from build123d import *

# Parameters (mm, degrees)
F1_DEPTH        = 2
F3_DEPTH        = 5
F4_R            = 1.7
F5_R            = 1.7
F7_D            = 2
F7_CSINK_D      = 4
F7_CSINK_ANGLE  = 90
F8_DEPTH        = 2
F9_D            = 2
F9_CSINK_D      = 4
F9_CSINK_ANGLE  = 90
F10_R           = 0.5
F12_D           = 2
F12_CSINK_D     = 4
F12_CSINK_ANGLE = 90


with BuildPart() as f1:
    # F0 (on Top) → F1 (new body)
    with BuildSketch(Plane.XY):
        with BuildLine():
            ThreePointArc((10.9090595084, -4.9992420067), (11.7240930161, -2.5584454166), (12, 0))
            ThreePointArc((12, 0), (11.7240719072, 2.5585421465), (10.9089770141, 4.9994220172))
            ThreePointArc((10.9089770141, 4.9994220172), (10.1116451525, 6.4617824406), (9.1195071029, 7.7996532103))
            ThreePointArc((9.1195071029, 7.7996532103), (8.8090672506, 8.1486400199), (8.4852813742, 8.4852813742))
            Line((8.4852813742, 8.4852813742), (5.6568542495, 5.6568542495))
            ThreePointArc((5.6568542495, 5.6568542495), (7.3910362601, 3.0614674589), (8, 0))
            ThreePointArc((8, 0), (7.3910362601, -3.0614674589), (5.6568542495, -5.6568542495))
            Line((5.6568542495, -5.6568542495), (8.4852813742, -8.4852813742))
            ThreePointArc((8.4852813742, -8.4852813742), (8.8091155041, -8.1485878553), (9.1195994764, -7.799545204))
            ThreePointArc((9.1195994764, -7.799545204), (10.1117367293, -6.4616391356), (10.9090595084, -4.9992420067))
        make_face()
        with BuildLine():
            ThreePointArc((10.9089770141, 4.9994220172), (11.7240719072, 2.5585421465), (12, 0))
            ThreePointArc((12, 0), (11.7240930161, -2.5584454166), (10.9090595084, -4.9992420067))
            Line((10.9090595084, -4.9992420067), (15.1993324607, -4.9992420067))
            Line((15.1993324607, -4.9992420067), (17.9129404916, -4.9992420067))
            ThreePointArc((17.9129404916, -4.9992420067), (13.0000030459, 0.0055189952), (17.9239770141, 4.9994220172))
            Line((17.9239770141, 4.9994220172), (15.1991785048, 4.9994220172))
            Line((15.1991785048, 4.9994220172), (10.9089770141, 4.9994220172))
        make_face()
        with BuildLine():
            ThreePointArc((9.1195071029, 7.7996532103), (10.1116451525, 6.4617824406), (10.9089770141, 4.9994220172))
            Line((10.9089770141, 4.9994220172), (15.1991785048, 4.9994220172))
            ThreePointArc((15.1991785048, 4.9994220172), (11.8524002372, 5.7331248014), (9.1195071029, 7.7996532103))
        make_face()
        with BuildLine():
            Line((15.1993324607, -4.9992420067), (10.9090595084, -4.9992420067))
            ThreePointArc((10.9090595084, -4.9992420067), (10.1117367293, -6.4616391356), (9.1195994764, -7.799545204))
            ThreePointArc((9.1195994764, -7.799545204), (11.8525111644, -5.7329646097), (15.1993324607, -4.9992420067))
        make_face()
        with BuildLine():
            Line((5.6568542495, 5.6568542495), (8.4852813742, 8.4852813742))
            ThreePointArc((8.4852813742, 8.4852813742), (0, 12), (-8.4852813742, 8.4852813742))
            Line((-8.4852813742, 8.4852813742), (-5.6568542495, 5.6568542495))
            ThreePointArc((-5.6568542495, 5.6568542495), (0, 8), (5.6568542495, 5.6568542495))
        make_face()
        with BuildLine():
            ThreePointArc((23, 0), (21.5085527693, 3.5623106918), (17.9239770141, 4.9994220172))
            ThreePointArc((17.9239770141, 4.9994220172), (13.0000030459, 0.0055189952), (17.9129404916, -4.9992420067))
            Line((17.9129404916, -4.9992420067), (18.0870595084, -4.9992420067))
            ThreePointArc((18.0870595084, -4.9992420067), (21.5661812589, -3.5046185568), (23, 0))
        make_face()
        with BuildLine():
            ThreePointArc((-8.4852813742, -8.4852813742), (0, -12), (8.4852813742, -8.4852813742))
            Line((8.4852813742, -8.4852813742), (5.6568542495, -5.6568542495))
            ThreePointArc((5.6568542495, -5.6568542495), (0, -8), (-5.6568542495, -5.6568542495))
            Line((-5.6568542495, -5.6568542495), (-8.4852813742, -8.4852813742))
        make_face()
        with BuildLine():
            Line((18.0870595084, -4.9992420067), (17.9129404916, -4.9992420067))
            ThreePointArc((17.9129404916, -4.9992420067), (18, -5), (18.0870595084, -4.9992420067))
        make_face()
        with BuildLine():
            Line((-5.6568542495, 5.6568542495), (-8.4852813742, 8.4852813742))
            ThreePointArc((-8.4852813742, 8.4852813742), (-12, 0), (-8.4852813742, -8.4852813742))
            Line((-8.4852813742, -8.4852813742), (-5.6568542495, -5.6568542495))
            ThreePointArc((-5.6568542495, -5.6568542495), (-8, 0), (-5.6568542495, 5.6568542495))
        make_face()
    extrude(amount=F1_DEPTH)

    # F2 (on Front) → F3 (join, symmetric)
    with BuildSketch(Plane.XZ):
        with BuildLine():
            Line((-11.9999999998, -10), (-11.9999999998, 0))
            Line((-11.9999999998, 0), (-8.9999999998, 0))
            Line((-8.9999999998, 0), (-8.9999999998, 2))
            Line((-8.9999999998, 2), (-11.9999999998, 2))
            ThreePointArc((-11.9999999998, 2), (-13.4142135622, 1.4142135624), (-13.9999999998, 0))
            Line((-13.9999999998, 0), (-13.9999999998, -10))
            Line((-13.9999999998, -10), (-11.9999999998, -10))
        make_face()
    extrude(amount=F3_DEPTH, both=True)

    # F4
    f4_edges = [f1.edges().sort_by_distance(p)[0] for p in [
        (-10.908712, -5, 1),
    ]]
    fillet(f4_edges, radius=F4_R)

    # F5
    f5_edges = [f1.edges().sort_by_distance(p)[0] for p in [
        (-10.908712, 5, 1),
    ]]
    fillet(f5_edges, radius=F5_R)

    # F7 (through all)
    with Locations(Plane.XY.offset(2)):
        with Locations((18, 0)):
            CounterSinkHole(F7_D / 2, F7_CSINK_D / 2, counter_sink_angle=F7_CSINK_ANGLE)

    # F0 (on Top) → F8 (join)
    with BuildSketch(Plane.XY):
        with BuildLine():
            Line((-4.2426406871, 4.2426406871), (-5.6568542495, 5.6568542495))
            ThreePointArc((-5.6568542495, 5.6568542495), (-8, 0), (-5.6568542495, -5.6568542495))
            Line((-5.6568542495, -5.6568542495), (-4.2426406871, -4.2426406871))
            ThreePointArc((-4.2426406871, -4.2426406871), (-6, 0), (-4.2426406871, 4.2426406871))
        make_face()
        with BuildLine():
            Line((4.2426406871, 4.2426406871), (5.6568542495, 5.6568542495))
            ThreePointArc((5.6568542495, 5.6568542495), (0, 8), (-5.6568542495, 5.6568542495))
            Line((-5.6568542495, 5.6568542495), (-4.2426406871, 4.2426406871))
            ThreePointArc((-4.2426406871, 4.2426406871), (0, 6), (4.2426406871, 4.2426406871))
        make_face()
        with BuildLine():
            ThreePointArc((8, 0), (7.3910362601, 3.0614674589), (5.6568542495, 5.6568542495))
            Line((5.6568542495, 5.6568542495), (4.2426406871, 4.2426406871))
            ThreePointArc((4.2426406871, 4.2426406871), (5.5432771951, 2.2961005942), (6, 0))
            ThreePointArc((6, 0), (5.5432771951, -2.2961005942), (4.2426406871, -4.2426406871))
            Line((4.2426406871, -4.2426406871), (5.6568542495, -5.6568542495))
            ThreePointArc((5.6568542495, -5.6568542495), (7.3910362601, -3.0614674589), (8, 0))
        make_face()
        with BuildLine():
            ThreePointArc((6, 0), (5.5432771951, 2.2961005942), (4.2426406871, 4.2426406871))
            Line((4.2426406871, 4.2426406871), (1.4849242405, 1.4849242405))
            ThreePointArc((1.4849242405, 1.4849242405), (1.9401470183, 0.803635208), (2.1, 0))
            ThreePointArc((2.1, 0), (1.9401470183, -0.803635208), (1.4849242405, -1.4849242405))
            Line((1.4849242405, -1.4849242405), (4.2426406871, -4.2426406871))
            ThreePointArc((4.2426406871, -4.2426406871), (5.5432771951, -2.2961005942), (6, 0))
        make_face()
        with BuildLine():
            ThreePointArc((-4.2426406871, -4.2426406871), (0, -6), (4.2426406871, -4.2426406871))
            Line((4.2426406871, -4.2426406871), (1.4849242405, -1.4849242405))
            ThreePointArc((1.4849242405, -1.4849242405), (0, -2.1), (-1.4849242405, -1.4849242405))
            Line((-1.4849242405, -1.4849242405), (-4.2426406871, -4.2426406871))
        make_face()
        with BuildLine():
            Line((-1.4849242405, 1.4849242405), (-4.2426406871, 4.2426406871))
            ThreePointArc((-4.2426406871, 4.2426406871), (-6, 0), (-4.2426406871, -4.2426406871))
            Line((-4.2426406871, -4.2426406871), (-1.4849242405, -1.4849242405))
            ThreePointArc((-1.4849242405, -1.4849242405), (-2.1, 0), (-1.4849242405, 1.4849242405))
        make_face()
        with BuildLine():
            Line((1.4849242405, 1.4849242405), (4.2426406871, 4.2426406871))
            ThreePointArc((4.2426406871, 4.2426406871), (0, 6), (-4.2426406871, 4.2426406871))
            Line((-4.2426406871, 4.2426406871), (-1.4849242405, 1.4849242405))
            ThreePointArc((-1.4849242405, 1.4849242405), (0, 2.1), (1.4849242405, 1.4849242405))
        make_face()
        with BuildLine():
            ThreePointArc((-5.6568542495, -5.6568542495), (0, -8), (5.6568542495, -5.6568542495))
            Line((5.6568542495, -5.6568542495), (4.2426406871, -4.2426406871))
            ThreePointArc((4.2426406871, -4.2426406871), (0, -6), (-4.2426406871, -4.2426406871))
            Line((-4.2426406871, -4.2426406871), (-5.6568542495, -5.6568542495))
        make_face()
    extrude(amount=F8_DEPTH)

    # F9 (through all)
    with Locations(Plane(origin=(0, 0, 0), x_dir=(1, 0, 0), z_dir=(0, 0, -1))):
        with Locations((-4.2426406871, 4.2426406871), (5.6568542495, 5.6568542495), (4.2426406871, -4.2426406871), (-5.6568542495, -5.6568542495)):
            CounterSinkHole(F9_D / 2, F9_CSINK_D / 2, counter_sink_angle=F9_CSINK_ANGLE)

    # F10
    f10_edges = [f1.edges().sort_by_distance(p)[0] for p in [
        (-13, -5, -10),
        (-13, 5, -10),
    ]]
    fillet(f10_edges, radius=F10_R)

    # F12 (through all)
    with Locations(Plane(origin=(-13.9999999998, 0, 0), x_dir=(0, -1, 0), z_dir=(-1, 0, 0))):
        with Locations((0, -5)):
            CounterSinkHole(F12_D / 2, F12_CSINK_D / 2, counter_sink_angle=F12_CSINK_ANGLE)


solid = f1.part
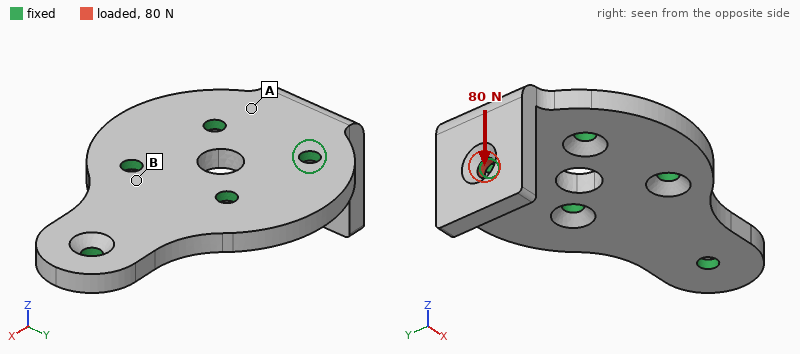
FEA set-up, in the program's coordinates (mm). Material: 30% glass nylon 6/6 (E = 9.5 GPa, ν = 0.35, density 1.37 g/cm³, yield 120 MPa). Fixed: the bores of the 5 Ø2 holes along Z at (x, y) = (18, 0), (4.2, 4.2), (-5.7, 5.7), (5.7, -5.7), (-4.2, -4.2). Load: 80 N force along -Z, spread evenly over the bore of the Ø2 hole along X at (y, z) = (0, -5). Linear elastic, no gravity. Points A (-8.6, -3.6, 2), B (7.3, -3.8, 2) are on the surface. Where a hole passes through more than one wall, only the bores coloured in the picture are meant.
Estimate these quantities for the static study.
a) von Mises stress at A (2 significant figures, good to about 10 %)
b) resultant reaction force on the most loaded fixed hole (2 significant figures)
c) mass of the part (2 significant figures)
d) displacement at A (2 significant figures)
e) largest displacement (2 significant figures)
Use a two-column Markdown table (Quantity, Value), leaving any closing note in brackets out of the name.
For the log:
| Quantity | Value |
|---|---|
| von Mises stress at A | 30 MPa |
| resultant reaction force on the most loaded fixed hole | 68 N |
| mass of the part | 1.7 g |
| displacement at A | 0.073 mm |
| largest displacement | 0.40 mm |
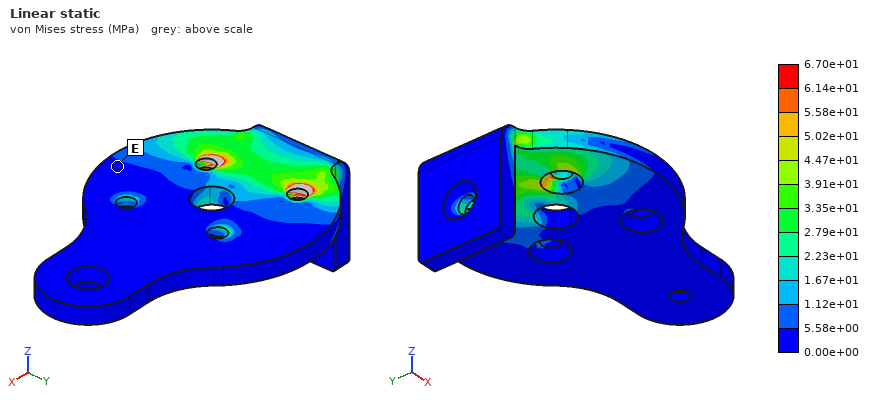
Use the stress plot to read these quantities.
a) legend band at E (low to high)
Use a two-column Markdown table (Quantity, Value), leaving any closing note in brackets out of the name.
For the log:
| Quantity | Value |
|---|---|
| legend band at E | 0.00e+00 to 5.58e+00 MPa |
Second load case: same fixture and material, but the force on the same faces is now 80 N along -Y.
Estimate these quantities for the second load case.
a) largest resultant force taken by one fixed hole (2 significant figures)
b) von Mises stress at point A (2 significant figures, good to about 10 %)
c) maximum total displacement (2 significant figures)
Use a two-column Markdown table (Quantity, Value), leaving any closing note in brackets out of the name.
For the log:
| Quantity | Value |
|---|---|
| largest resultant force taken by one fixed hole | 88 N |
| von Mises stress at point A | 24 MPa |
| maximum total displacement | 0.27 mm |
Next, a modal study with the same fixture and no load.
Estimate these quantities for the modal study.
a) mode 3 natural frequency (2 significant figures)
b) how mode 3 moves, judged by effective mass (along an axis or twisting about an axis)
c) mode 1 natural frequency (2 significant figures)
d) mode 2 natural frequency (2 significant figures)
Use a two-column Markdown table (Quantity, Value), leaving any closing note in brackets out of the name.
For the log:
| Quantity | Value |
|---|---|
| mode 3 natural frequency | 8800 Hz |
| how mode 3 moves, judged by effective mass | along Z |
| mode 1 natural frequency | 3400 Hz |
| mode 2 natural frequency | 6300 Hz |
